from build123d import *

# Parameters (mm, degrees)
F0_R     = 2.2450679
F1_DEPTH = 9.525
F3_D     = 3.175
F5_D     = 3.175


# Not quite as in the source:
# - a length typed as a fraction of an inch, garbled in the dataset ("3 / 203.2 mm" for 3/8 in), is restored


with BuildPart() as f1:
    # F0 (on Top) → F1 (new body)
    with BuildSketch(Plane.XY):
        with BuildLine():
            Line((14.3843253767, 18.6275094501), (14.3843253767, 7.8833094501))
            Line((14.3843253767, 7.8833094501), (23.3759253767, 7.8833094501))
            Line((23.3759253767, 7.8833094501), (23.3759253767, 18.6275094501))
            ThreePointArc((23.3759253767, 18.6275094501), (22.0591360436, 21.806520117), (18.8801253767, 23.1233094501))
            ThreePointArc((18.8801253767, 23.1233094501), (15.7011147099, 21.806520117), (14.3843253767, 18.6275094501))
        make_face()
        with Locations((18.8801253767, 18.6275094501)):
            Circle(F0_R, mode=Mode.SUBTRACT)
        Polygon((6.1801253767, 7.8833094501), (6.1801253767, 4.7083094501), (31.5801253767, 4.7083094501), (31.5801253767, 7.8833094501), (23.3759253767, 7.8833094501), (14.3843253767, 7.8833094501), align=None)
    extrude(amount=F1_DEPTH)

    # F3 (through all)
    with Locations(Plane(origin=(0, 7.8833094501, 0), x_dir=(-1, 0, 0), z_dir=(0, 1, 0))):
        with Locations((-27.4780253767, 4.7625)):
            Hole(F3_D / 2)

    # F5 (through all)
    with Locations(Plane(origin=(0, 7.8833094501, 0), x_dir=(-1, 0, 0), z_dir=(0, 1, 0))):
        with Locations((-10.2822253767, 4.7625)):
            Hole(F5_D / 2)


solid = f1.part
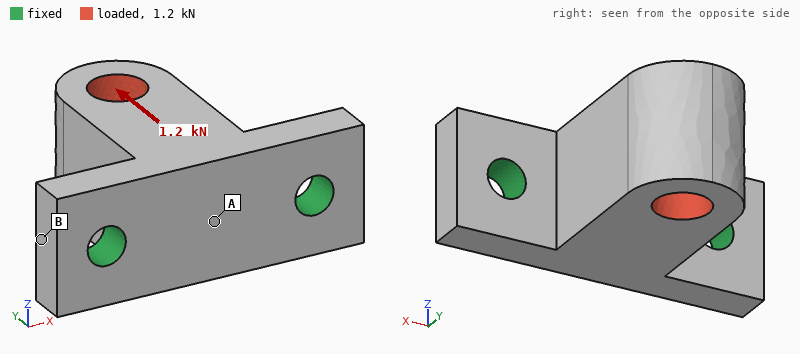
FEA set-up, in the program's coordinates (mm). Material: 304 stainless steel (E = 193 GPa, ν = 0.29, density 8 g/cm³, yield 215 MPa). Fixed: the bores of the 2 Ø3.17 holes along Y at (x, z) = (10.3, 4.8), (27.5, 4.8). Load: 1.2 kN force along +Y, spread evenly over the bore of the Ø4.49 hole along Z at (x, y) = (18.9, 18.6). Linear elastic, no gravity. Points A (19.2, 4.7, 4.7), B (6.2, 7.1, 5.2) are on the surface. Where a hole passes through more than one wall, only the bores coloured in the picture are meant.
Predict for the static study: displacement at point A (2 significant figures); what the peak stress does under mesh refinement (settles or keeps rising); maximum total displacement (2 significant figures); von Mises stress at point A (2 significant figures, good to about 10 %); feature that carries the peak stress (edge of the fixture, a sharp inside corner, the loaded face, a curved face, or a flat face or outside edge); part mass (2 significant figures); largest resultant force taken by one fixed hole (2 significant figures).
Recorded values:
2.9 µm
keeps rising
4.3 µm
28 MPa
edge of the fixture
14 g
630 N
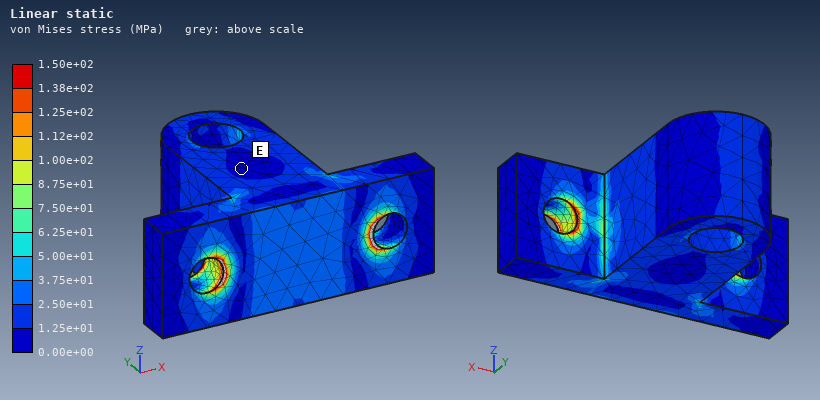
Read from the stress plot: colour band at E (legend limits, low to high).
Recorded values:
0.00e+00 to 1.25e+01 MPa
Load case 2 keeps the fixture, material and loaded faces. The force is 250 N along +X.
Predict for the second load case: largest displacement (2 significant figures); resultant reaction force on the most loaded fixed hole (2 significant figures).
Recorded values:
5.4 µm
270 N
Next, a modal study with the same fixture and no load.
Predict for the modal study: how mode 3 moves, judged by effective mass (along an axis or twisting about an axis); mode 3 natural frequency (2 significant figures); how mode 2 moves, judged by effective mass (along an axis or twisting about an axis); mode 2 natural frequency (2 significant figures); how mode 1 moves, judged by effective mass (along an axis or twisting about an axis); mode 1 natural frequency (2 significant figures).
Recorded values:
along Y
30 kHz
along X
18 kHz
along Z
9800 Hz
